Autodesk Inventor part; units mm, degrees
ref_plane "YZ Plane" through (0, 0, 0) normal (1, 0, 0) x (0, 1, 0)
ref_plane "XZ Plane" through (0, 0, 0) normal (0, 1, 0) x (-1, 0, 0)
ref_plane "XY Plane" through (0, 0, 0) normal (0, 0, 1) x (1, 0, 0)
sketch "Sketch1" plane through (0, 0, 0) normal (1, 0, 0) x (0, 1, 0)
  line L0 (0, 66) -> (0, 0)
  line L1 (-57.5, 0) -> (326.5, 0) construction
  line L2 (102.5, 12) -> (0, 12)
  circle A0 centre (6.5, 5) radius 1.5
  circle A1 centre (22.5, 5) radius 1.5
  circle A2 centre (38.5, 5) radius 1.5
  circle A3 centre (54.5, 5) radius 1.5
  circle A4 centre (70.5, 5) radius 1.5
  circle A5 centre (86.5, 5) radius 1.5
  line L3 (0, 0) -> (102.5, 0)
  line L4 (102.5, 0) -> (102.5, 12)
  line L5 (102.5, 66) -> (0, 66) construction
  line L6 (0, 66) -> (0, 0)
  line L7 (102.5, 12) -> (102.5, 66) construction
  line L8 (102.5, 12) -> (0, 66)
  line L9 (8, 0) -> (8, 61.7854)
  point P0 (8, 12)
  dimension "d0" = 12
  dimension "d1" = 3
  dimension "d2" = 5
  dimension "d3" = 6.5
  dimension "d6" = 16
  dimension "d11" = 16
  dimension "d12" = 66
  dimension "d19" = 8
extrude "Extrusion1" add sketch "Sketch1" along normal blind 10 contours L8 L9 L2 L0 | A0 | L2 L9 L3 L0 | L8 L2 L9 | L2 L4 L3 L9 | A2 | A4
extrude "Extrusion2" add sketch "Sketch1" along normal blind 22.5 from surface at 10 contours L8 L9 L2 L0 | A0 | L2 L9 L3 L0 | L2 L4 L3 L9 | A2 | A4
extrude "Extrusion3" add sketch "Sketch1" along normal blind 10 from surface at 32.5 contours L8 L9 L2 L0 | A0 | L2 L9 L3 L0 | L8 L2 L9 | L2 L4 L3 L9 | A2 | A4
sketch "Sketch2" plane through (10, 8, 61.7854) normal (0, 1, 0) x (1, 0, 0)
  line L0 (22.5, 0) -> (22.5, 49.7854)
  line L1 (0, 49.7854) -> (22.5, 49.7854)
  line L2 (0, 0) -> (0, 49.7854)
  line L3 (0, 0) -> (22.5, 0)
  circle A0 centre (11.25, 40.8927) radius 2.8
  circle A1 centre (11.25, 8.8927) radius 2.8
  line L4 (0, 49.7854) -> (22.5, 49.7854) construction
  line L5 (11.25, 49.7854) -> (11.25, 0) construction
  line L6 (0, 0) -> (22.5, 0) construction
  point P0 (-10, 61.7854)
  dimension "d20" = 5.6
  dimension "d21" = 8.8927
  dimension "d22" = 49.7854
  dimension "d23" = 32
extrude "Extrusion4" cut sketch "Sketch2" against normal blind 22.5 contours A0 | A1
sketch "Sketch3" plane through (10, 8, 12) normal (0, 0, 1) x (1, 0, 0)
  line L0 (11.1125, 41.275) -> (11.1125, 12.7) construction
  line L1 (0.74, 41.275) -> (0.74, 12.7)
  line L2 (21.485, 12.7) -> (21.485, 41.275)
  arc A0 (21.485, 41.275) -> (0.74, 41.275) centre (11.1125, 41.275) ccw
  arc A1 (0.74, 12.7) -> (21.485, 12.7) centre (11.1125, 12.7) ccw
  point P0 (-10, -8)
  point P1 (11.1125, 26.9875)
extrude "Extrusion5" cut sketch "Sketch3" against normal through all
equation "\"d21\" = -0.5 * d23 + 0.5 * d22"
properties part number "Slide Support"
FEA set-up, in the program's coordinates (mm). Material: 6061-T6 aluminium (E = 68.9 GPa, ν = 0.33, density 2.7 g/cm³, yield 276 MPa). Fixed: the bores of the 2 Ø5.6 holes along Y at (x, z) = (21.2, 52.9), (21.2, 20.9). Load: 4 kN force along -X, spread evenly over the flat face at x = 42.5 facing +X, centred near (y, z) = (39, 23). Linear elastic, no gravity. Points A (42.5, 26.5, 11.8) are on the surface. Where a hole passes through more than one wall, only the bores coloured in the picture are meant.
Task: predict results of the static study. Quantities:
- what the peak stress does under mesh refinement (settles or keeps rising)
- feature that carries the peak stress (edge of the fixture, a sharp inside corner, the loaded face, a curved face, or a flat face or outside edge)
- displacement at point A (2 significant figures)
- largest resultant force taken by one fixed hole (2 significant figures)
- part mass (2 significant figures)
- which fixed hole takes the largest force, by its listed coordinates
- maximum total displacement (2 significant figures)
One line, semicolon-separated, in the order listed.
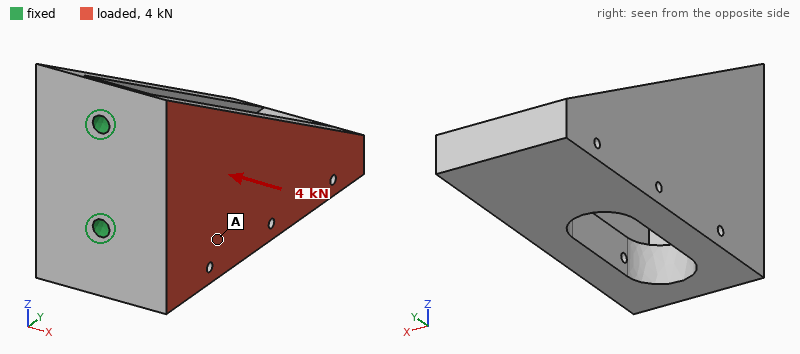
keeps rising; edge of the fixture; 0.19 mm; 3.5 kN; 280 g; (21.2, 20.9); 0.59 mm
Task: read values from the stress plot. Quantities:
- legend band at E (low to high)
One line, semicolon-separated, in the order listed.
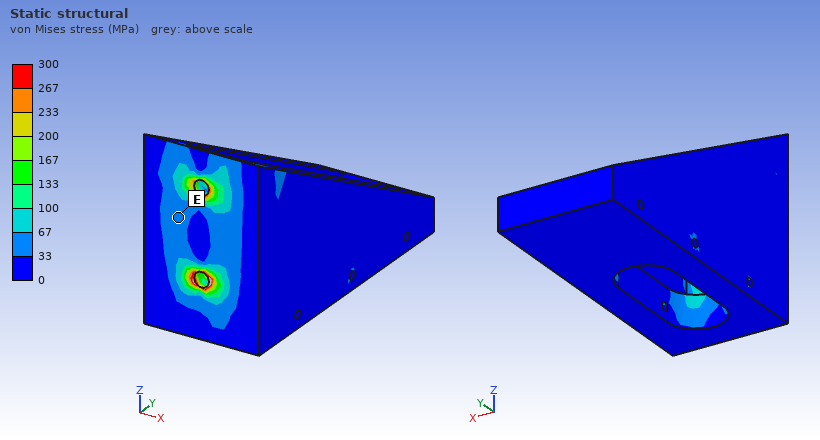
33 to 67 MPa
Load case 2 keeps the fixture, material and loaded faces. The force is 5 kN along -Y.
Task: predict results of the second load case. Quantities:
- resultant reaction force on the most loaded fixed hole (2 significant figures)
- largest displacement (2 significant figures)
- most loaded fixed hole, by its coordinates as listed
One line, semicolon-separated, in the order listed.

4.3 kN; 0.38 mm; (21.2, 20.9)
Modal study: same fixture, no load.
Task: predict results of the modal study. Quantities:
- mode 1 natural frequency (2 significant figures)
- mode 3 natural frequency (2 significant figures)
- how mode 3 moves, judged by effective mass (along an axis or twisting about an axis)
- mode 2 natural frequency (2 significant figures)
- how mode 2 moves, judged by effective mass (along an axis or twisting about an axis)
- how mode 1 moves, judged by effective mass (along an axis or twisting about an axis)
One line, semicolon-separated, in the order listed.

950 Hz; 4500 Hz; twisting about Y; 2000 Hz; along Z; along X
